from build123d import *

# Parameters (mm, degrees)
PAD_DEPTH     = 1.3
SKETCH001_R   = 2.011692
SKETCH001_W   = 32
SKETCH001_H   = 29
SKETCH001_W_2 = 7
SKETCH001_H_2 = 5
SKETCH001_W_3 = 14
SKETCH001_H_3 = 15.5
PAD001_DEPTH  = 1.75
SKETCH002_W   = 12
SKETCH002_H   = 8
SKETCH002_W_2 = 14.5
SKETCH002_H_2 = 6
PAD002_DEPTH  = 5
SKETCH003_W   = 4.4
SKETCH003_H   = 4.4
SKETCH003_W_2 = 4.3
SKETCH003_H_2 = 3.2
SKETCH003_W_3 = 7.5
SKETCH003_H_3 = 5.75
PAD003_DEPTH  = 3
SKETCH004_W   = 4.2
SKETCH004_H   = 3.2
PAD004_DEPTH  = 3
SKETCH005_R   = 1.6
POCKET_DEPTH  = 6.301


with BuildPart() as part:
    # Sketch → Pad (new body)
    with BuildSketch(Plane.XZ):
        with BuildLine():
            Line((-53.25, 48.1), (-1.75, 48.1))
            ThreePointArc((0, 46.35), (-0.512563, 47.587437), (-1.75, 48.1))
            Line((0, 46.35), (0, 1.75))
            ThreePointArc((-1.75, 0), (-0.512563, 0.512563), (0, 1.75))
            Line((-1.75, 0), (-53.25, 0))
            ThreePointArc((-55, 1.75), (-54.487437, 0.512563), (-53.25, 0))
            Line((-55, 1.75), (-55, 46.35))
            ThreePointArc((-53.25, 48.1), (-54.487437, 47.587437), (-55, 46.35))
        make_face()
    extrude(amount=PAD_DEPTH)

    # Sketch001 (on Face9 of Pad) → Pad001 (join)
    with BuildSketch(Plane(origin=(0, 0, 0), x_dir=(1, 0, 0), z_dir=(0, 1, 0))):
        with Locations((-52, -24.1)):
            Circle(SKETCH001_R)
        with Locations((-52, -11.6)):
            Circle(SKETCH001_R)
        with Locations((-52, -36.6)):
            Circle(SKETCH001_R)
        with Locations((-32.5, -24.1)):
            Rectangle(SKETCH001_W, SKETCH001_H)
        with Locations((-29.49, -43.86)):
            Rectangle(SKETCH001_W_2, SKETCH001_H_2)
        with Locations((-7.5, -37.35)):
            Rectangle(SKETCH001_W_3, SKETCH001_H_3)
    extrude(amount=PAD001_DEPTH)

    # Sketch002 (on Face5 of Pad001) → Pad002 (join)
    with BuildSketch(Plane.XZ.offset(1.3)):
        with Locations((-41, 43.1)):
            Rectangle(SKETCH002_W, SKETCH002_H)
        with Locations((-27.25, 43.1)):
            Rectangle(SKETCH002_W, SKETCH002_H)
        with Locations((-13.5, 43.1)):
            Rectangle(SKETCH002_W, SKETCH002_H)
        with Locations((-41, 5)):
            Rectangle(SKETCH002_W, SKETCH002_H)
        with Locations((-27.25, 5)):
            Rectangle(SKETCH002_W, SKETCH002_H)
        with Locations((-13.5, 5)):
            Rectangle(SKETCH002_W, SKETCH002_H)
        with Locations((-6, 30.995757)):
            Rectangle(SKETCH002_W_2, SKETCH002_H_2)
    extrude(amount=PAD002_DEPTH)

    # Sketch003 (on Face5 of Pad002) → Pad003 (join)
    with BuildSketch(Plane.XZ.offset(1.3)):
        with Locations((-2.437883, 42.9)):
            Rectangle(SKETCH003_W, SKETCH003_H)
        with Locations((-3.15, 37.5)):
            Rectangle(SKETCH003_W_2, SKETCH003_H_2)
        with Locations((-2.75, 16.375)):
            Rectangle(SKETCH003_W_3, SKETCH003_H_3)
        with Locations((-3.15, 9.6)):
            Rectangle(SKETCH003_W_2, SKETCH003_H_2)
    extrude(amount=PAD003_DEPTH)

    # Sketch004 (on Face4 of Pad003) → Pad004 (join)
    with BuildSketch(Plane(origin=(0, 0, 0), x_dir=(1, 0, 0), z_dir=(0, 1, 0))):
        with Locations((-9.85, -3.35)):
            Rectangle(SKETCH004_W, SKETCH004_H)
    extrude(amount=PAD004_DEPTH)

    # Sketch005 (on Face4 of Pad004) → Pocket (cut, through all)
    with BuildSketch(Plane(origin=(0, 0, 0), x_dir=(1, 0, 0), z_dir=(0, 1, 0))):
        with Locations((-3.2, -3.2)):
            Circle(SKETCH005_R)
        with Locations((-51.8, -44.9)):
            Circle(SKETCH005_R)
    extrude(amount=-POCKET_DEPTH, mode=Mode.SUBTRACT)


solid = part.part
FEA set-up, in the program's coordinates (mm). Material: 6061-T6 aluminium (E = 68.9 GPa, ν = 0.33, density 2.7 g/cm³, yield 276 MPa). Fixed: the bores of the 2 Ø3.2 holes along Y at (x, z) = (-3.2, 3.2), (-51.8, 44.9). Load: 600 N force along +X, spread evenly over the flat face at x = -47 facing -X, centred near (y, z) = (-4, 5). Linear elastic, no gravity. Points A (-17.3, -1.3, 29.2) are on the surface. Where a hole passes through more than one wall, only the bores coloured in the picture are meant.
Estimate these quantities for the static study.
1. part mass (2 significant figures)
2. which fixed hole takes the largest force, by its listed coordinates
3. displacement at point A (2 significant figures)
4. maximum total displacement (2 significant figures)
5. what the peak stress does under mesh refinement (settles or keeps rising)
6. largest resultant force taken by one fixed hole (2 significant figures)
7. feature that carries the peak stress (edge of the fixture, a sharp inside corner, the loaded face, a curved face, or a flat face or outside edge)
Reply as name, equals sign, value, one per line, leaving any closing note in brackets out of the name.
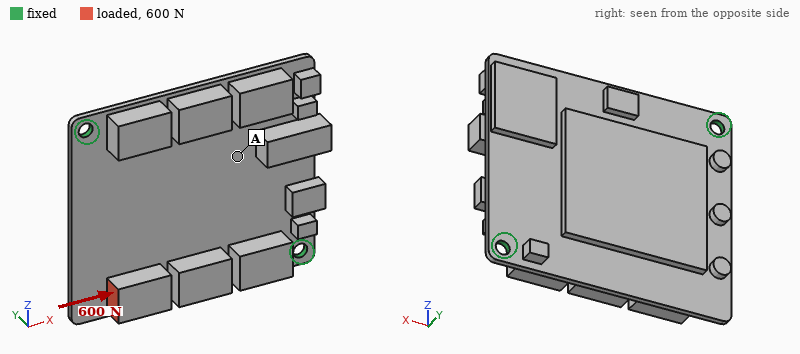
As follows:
part mass = 25 g
which fixed hole takes the largest force, by its listed coordinates = (-3.2, 3.2)
displacement at point A = 0.10 mm
maximum total displacement = 0.52 mm
what the peak stress does under mesh refinement = keeps rising
largest resultant force taken by one fixed hole = 500 N
feature that carries the peak stress = edge of the fixture
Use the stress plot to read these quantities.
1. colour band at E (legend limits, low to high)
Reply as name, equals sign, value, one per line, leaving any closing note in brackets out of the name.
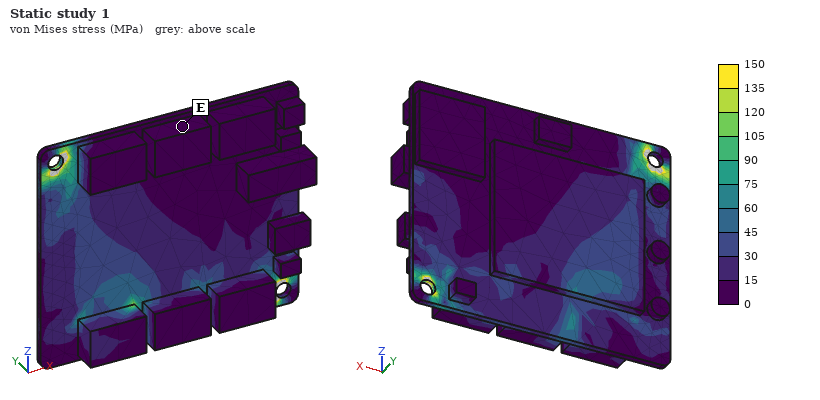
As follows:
colour band at E = 0 to 15 MPa
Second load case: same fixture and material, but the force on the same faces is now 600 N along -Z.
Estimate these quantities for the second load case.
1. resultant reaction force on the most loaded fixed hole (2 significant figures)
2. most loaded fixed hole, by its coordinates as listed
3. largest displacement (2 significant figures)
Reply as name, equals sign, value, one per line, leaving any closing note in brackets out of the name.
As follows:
resultant reaction force on the most loaded fixed hole = 460 N
most loaded fixed hole, by its coordinates as listed = (-51.8, 44.9)
largest displacement = 0.46 mm
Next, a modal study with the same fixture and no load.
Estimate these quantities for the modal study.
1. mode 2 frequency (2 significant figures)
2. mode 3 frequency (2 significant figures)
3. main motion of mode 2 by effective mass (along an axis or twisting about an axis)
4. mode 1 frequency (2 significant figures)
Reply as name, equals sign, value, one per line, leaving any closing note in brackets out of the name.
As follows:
mode 2 frequency = 1300 Hz
mode 3 frequency = 3600 Hz
main motion of mode 2 by effective mass = along Y
mode 1 frequency = 720 Hz
